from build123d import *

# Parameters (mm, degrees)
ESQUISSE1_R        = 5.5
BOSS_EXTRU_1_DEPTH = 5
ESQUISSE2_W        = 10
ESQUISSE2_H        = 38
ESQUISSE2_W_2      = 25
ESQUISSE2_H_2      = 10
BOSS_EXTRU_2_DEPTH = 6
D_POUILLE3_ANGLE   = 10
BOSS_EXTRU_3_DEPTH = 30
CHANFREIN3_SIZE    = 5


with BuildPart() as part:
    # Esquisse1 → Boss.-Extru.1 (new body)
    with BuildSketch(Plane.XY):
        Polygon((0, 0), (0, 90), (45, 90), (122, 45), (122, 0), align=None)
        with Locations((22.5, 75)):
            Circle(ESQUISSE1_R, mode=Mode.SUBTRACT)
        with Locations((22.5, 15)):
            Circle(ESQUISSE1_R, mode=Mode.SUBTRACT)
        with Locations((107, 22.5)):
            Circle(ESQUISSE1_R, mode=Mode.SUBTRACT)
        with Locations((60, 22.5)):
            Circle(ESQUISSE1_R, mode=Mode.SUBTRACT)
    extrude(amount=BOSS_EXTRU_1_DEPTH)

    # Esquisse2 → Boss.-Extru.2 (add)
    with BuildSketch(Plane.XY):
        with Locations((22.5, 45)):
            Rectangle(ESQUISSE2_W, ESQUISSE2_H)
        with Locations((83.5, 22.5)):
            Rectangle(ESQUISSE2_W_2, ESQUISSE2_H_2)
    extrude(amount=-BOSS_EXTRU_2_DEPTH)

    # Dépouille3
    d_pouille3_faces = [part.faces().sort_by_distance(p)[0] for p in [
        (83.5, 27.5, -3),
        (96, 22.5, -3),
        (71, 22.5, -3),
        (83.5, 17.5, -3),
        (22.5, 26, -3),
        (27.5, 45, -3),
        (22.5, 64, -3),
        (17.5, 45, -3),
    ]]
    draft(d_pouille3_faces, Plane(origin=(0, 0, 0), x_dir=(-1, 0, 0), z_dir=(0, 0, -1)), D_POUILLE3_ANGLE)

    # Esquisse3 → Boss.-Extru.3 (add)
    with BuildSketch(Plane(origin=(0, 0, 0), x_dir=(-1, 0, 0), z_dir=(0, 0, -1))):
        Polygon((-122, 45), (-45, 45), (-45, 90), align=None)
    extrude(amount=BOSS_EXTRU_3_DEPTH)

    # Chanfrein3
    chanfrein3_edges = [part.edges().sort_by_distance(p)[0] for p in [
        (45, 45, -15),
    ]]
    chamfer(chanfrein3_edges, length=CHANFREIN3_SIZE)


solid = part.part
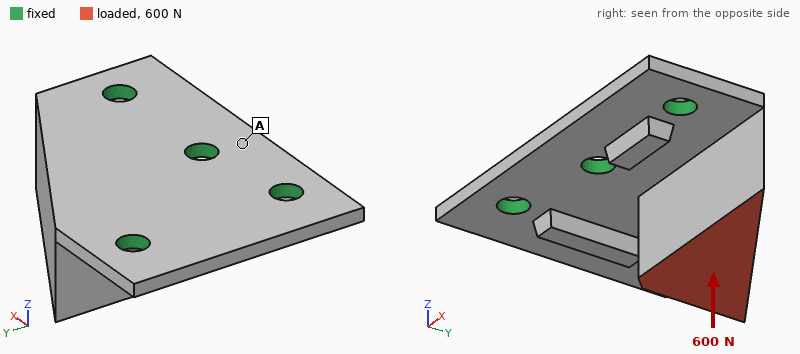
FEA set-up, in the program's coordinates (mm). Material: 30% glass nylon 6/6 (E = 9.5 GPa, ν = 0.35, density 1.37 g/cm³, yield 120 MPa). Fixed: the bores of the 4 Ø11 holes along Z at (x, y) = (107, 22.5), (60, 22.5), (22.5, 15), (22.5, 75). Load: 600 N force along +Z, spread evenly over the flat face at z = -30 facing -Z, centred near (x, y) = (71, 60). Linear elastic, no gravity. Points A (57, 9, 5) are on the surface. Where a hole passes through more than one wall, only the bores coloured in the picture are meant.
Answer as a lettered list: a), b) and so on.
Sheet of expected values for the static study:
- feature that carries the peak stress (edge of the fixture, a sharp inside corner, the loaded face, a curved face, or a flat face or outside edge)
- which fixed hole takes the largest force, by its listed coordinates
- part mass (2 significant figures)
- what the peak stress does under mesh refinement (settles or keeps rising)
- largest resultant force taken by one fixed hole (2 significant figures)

a) edge of the fixture
b) (22.5, 75)
c) 140 g
d) keeps rising
e) 340 N
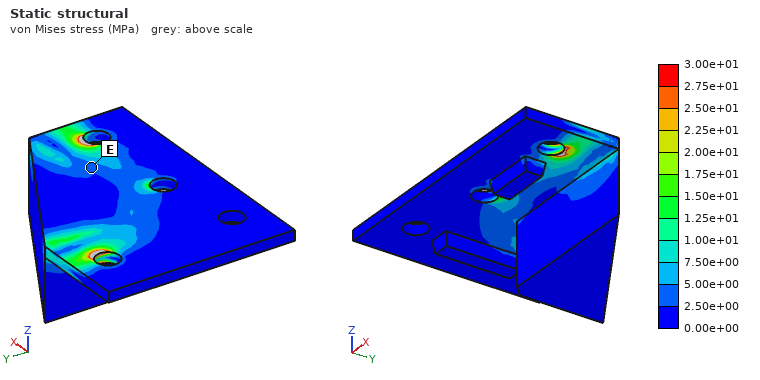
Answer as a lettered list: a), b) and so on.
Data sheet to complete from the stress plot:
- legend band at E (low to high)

a) 2.50e+00 to 5.00e+00 MPa
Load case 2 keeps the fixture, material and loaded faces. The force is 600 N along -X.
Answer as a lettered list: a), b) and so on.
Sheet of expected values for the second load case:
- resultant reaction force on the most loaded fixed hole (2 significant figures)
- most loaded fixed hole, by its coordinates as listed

a) 400 N
b) (107, 22.5)
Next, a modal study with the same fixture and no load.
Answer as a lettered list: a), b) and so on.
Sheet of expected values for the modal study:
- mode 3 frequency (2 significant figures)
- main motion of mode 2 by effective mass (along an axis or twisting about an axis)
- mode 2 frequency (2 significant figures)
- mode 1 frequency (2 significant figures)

a) 2200 Hz
b) along X
c) 2100 Hz
d) 960 Hz
